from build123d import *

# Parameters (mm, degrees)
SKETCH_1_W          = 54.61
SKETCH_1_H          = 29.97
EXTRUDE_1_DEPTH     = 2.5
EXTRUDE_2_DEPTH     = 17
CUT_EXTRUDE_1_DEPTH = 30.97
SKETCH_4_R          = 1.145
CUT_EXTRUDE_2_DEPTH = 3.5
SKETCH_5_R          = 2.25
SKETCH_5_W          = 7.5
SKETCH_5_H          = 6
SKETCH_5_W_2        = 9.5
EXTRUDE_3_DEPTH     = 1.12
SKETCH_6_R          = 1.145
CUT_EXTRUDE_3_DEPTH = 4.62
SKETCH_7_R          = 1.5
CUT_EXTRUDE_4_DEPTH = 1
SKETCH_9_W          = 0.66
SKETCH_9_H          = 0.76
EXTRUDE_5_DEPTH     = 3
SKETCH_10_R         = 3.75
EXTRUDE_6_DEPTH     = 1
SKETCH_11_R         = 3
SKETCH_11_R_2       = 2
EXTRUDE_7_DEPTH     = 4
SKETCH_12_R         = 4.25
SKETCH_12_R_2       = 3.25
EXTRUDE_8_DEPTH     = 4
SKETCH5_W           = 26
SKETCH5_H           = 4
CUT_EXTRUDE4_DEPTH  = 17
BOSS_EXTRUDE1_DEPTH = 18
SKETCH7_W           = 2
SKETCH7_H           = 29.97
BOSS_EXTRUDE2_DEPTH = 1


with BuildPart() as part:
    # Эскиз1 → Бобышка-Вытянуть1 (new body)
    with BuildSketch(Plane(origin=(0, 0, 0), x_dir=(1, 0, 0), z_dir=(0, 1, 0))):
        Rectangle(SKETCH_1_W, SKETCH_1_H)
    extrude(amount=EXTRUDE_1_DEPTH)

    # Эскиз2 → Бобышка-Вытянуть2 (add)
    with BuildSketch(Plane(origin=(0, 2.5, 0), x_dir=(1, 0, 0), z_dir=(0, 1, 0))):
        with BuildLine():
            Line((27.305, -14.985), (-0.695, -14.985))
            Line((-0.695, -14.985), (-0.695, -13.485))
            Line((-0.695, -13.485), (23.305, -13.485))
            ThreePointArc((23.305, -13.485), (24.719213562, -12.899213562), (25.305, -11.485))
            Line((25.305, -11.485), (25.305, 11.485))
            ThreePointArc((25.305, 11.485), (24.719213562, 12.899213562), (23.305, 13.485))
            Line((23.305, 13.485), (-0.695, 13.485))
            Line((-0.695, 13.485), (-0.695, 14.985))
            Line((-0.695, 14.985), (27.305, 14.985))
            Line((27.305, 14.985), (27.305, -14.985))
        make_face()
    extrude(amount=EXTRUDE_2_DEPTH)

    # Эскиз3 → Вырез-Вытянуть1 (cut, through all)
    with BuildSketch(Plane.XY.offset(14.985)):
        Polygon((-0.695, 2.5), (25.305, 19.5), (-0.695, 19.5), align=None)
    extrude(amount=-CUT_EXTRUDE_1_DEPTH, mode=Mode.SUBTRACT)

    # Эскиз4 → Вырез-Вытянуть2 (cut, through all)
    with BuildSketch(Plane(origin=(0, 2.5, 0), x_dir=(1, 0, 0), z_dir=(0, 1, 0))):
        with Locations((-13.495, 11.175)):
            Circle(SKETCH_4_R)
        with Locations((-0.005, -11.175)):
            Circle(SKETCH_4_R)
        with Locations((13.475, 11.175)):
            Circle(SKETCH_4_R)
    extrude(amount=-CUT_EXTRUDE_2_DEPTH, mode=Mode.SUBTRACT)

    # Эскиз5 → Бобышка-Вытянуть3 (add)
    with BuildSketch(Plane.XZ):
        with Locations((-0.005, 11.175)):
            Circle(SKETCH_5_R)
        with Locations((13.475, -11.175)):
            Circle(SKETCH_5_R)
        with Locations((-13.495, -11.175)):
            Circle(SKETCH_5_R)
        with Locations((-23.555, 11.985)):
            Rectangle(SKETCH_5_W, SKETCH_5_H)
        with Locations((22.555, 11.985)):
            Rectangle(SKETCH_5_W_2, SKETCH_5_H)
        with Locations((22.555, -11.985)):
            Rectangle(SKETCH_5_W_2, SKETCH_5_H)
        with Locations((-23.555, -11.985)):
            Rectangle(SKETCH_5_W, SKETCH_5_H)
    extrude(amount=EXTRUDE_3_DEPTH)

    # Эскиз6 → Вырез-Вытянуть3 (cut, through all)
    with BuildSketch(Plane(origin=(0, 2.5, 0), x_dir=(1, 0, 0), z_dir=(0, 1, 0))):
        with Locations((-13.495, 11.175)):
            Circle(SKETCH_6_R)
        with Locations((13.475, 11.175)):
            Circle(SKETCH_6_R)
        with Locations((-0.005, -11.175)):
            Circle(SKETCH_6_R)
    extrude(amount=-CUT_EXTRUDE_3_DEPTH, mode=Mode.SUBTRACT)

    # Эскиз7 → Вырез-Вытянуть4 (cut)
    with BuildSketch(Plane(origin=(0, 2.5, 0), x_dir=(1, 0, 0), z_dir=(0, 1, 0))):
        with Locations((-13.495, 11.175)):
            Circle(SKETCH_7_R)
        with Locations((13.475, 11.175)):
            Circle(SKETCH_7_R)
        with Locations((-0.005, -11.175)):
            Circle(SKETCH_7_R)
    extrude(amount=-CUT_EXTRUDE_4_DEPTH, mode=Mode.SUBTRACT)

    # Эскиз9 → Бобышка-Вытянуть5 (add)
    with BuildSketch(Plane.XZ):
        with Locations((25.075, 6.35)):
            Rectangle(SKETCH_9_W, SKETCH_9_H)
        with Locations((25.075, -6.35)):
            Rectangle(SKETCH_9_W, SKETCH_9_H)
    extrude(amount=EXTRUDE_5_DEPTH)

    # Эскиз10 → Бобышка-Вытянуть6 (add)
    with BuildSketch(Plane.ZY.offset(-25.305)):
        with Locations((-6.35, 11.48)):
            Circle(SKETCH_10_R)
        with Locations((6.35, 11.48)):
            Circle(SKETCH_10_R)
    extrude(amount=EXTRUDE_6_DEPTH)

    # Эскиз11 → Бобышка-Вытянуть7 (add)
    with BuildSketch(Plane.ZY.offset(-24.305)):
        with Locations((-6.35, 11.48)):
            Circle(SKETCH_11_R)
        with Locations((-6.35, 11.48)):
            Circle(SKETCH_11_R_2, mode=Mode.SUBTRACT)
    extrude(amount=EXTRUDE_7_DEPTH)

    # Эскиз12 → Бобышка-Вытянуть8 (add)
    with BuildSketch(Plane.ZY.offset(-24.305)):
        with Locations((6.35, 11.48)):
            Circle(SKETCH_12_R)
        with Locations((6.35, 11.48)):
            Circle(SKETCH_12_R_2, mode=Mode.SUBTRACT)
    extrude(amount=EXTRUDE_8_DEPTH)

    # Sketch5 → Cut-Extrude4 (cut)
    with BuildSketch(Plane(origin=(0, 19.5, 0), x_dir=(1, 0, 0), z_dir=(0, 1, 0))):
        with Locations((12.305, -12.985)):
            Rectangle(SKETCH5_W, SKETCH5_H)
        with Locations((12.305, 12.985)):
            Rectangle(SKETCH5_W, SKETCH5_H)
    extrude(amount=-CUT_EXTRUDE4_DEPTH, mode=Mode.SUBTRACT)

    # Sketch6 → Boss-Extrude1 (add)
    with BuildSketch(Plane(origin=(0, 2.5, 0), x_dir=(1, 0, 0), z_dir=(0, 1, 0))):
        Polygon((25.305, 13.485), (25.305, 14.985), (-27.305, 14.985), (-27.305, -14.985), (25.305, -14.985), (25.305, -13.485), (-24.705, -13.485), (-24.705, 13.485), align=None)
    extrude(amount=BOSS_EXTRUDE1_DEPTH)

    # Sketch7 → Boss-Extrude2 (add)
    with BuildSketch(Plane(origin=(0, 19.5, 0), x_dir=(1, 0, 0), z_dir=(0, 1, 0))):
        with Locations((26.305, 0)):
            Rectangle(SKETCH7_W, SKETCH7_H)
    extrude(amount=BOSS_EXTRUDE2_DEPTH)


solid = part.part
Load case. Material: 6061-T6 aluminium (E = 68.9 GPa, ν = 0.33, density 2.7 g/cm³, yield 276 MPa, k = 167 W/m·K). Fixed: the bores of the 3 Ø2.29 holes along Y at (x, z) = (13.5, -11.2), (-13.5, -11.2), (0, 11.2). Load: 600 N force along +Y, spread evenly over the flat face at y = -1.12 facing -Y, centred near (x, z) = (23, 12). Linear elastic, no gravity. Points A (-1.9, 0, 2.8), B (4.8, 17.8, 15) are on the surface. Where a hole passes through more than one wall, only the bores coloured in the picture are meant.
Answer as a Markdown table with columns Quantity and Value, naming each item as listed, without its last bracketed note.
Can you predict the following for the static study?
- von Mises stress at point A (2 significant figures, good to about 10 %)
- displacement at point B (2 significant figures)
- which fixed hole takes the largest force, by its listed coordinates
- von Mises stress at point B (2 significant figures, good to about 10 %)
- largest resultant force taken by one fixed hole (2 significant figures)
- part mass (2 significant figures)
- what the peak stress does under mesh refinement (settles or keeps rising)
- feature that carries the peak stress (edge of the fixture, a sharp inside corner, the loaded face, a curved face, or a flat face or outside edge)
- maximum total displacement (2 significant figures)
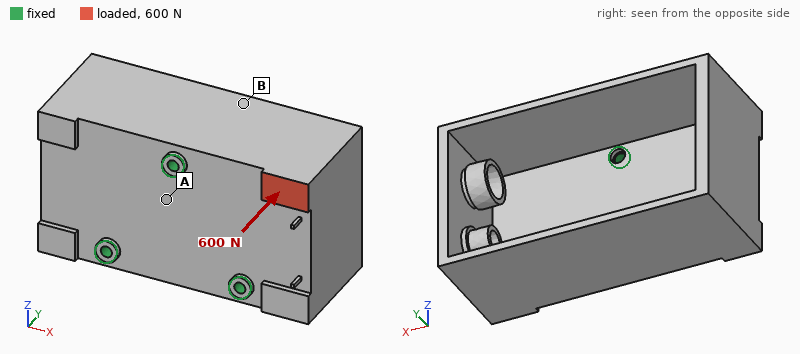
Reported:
| Quantity | Value |
|---|---|
| von Mises stress at point A | 21 MPa |
| displacement at point B | 0.17 mm |
| which fixed hole takes the largest force, by its listed coordinates | (0, 11.2) |
| von Mises stress at point B | 55 MPa |
| largest resultant force taken by one fixed hole | 630 N |
| part mass | 26 g |
| what the peak stress does under mesh refinement | keeps rising |
| feature that carries the peak stress | edge of the fixture |
| maximum total displacement | 0.38 mm |
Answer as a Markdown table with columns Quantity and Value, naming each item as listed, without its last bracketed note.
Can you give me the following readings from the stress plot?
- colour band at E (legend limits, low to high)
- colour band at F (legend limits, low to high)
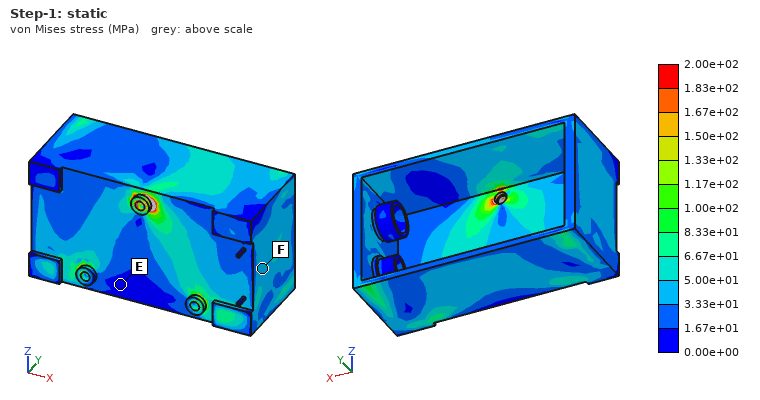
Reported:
| Quantity | Value |
|---|---|
| colour band at E | 0.00e+00 to 1.67e+01 MPa |
| colour band at F | 3.33e+01 to 5.00e+01 MPa |
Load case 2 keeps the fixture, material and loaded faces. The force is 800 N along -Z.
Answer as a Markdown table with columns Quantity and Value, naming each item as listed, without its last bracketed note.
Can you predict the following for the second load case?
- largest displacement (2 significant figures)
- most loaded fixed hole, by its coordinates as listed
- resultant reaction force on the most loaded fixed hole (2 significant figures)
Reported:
| Quantity | Value |
|---|---|
| largest displacement | 47 µm |
| most loaded fixed hole, by its coordinates as listed | (13.5, -11.2) |
| resultant reaction force on the most loaded fixed hole | 730 N |
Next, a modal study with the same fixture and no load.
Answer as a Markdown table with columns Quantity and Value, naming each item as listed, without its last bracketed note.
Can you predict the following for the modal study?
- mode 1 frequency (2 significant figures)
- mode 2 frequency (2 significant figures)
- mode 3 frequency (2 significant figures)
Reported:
| Quantity | Value |
|---|---|
| mode 1 frequency | 2500 Hz |
| mode 2 frequency | 4900 Hz |
| mode 3 frequency | 5100 Hz |
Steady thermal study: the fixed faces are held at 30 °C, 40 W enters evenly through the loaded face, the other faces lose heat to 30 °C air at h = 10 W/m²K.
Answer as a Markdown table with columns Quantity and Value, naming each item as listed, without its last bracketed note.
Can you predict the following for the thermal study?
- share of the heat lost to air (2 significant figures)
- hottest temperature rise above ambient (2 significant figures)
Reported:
| Quantity | Value |
|---|---|
| share of the heat lost to air | 4.3 % |
| hottest temperature rise above ambient | 75 K |
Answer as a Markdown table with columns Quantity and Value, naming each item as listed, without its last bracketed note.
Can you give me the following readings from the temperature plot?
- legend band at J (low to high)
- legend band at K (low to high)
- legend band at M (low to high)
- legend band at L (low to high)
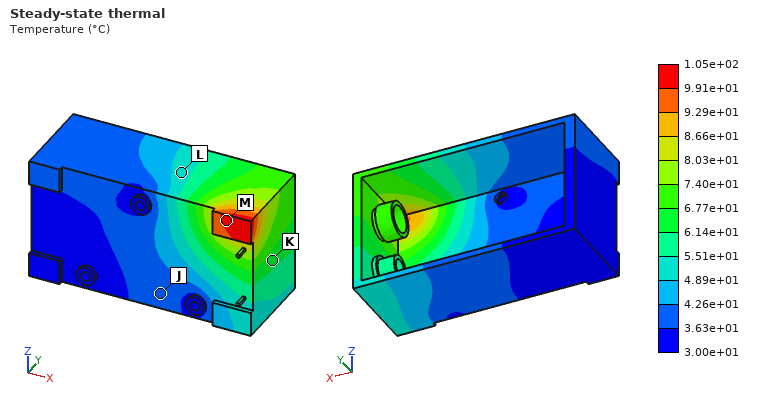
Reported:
| Quantity | Value |
|---|---|
| legend band at J | 3.63e+01 to 4.26e+01 °C |
| legend band at K | 6.14e+01 to 6.77e+01 °C |
| legend band at M | 9.91e+01 to 1.05e+02 °C |
| legend band at L | 4.89e+01 to 5.51e+01 °C |
